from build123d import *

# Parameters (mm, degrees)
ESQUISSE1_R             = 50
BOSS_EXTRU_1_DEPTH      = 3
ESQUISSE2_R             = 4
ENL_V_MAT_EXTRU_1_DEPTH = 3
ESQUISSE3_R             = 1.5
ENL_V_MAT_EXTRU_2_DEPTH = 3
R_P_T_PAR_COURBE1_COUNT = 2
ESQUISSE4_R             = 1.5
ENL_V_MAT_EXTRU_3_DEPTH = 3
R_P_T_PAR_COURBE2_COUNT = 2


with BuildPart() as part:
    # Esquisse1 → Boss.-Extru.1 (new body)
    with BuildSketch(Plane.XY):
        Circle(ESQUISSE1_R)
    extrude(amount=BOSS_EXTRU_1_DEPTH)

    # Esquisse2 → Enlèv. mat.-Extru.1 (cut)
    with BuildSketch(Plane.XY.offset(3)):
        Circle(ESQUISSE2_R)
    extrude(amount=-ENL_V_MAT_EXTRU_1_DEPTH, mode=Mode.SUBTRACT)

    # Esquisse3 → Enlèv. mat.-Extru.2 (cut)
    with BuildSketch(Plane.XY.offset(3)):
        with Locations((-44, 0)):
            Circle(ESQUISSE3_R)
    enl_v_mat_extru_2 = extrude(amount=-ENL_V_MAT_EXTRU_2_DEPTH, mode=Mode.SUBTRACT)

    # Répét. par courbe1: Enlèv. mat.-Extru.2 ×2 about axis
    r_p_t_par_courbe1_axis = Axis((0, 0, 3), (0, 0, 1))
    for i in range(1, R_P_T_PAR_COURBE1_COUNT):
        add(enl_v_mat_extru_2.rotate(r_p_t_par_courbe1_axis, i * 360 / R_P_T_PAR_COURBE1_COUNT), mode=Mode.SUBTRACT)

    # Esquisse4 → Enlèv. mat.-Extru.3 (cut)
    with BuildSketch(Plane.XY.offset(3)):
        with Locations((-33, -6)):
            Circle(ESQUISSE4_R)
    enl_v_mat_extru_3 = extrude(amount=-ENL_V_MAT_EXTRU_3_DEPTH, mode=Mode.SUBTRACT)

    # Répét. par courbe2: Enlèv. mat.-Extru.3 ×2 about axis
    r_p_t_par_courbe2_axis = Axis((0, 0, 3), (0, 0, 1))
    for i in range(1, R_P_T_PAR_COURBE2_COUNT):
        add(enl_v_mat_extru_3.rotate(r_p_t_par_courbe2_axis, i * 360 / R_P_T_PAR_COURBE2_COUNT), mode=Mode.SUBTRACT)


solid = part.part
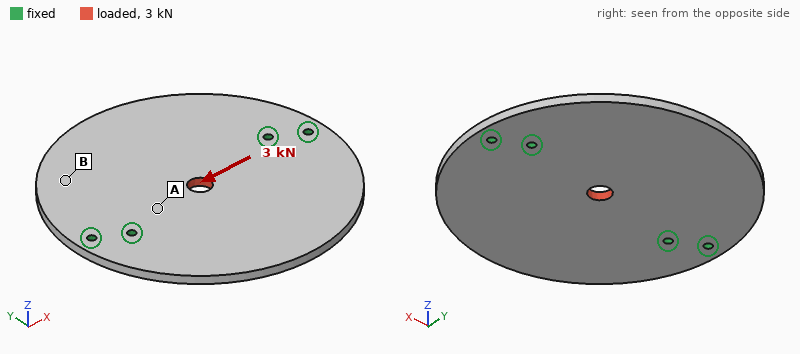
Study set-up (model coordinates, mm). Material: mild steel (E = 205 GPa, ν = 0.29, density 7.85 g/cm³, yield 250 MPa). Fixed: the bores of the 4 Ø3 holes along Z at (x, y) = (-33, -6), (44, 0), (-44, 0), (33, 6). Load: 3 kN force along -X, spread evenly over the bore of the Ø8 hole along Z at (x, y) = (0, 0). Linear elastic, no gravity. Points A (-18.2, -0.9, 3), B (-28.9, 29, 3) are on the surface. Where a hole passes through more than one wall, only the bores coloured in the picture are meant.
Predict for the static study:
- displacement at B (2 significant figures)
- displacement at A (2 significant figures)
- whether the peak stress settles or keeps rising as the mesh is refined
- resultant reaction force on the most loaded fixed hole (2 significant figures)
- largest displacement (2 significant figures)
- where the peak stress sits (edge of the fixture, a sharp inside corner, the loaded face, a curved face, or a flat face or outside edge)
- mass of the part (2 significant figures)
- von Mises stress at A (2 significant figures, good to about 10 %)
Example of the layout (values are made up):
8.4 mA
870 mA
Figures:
1.9 µm
2.0 µm
keeps rising
1.0 kN
4.0 µm
edge of the fixture
180 g
23 MPa
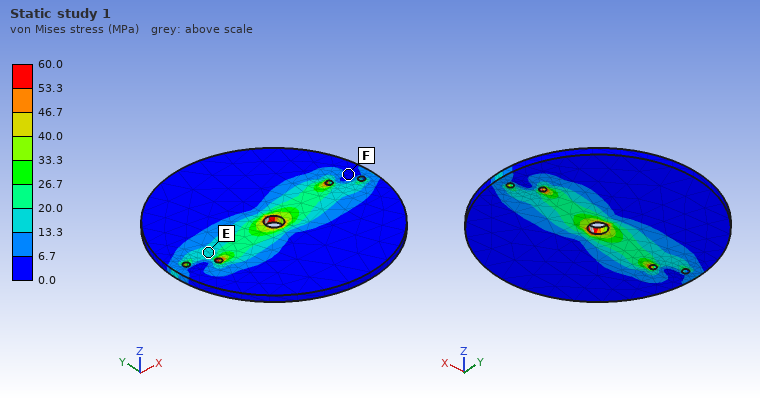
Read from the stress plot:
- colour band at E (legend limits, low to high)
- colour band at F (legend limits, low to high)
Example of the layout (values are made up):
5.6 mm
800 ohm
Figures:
13.3 to 20.0 MPa
0.0 to 6.7 MPa
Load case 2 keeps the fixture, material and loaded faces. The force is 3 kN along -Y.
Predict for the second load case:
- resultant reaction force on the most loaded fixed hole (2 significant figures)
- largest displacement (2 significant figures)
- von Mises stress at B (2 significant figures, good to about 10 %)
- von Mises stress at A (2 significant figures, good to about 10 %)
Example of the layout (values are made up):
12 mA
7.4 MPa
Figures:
1.1 kN
5.4 µm
7.9 MPa
11 MPa
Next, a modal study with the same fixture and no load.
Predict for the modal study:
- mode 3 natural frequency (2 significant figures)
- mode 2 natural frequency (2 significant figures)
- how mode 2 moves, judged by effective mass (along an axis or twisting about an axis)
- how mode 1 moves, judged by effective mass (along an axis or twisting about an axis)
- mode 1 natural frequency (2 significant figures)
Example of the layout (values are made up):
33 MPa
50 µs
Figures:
2700 Hz
1200 Hz
along Z
twisting about X
990 Hz
